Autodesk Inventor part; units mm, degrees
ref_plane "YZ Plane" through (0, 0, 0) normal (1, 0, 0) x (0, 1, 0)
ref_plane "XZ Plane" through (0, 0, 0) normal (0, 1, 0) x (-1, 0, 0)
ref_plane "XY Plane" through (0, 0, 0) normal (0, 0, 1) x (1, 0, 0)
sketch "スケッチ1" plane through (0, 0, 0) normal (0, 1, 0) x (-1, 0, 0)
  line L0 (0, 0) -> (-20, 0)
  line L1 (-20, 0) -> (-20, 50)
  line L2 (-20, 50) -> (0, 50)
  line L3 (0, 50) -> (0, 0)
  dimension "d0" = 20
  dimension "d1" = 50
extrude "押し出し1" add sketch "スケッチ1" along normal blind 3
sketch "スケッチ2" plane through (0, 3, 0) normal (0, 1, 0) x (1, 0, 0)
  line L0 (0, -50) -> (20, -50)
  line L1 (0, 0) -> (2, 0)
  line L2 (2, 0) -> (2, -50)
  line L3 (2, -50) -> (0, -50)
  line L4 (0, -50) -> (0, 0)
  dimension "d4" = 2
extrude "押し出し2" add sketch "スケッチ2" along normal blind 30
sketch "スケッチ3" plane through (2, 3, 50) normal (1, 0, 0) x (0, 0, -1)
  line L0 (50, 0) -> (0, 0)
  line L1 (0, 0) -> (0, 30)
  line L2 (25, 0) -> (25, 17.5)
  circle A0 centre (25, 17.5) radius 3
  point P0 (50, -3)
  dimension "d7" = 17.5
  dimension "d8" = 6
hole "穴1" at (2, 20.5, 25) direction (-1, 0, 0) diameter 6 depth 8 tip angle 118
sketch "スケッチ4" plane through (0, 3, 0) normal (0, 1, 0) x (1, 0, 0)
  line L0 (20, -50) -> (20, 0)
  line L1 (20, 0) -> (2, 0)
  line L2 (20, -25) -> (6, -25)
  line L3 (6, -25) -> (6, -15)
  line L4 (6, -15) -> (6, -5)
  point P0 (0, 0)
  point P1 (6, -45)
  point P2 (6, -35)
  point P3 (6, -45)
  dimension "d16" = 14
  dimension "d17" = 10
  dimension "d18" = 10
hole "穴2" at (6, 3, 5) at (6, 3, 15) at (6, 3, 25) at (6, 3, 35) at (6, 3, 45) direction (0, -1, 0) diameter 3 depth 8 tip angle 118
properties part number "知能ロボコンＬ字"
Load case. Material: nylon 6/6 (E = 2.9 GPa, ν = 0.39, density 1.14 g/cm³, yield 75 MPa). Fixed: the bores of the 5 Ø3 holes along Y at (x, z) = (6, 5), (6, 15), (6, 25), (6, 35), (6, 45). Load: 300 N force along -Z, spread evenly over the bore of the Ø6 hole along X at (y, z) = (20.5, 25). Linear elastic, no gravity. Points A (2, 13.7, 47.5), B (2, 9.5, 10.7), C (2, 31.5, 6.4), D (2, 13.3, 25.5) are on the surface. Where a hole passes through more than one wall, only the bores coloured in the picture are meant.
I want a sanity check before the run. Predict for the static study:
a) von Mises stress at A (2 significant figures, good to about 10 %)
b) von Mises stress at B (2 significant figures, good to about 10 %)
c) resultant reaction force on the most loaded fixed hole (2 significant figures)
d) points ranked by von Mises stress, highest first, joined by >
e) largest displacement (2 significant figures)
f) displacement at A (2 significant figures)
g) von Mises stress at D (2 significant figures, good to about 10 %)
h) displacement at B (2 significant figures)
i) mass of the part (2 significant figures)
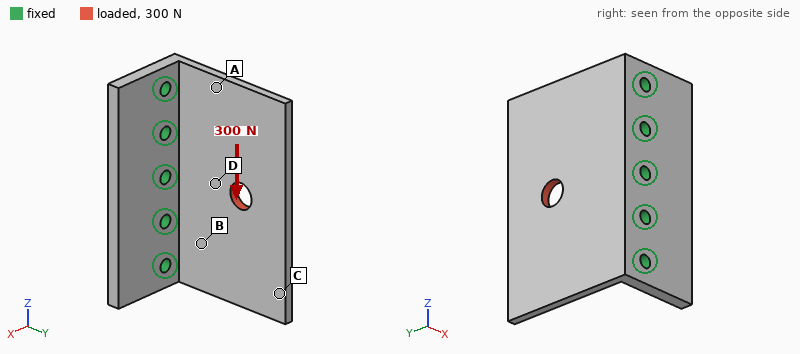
4.2 MPa
7.8 MPa
130 N
D > B > A > C
0.34 mm
0.19 mm
10 MPa
0.098 mm
6.7 g
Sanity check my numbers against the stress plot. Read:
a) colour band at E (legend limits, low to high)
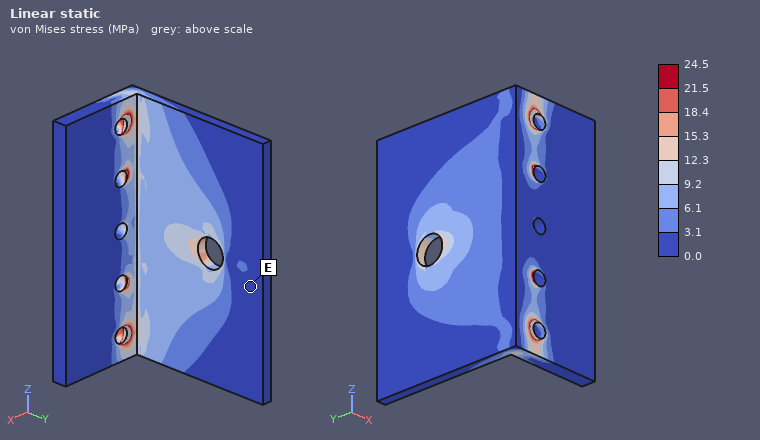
0.0 to 3.1 MPa
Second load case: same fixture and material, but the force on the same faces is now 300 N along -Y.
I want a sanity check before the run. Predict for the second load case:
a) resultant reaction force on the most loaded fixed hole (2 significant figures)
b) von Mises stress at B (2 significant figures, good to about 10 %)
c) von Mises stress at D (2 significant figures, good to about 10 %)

72 N
3.1 MPa
6.9 MPa
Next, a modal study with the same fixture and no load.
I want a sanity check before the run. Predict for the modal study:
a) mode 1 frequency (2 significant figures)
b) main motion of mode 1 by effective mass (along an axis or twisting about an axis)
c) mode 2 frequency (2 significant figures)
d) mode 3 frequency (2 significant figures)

530 Hz
along X
890 Hz
2000 Hz
